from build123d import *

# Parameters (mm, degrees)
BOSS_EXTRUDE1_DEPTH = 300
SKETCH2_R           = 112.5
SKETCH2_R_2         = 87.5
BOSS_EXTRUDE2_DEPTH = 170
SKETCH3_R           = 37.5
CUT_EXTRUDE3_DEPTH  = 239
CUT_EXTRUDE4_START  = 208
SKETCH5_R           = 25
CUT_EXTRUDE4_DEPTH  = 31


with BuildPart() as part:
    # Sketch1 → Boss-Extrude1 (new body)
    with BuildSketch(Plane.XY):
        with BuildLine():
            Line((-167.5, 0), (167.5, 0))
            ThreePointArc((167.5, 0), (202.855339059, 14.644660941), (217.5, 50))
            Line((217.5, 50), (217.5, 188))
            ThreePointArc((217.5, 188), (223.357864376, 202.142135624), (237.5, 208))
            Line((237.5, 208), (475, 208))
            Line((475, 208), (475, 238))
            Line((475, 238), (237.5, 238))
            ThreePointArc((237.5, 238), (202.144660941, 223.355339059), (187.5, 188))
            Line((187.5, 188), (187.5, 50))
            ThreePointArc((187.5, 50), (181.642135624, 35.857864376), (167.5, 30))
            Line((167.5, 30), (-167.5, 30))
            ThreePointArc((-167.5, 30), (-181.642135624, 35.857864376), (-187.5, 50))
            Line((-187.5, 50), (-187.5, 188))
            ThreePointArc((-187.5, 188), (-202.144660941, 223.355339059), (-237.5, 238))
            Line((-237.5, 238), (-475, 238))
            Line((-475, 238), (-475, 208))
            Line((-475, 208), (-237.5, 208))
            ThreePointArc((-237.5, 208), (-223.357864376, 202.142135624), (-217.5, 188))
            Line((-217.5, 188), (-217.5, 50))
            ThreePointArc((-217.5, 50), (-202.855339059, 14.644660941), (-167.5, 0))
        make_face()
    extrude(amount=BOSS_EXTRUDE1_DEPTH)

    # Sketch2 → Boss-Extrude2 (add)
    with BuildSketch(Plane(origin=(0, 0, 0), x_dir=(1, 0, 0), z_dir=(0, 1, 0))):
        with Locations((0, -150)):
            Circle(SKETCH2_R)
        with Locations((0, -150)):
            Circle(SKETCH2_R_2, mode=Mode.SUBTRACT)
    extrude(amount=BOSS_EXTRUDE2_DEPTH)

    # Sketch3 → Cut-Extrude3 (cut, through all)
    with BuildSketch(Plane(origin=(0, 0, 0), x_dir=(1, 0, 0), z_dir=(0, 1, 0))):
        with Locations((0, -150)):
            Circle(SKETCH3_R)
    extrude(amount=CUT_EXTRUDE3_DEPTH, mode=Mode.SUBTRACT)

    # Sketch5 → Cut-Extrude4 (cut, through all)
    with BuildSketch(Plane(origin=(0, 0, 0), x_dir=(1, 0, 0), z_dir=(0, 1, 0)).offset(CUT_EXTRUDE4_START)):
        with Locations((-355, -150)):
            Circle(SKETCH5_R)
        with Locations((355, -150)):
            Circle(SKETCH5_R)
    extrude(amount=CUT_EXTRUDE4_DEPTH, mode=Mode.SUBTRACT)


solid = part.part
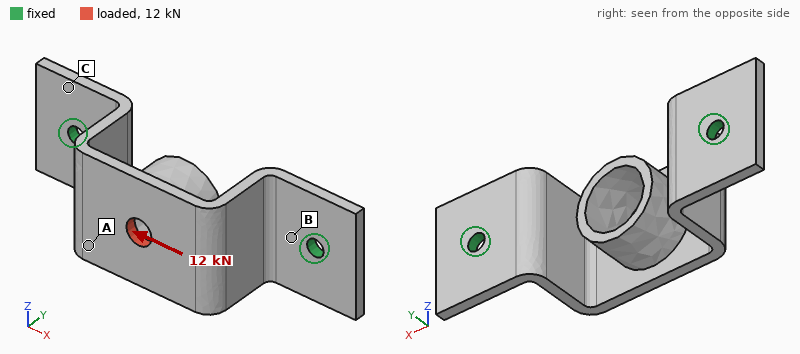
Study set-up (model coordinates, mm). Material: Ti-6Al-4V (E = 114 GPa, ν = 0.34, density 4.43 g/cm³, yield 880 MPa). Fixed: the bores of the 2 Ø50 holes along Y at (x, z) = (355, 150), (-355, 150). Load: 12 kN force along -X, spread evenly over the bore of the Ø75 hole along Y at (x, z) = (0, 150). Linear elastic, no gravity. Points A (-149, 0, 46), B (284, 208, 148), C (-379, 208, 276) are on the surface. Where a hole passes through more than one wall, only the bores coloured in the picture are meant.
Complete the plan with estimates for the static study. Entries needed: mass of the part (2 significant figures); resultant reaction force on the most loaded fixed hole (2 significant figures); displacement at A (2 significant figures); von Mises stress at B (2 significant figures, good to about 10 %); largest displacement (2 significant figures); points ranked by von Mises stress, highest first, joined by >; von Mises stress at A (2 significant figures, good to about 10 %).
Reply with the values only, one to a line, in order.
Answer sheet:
61 kg
6.9 kN
0.13 mm
7.0 MPa
0.18 mm
A > B > C
8.8 MPa
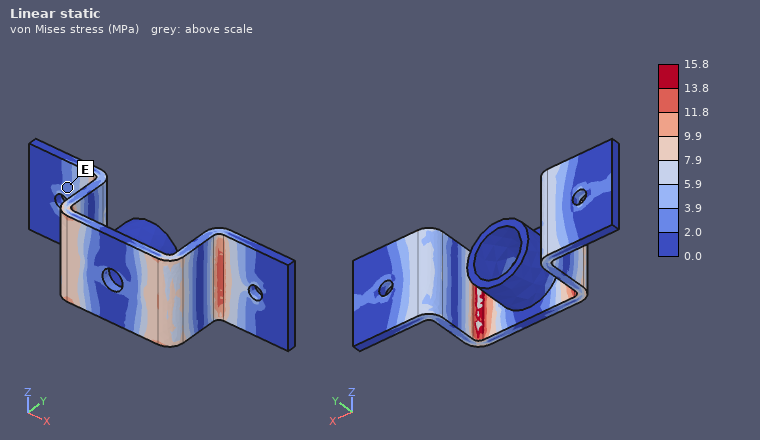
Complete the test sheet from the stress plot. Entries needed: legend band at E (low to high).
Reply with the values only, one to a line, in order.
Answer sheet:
2.0 to 3.9 MPa
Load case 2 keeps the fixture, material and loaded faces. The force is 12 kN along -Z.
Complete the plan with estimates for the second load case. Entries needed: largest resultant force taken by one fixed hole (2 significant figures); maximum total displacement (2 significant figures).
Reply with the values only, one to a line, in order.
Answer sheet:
6.0 kN
0.35 mm
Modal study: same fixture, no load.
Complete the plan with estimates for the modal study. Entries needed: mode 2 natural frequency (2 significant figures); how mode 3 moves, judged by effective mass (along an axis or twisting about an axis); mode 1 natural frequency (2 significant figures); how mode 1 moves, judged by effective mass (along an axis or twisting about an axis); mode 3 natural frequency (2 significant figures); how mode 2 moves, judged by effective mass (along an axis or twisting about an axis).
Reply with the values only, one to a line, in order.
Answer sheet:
250 Hz
along Y
190 Hz
along Z
400 Hz
along X
